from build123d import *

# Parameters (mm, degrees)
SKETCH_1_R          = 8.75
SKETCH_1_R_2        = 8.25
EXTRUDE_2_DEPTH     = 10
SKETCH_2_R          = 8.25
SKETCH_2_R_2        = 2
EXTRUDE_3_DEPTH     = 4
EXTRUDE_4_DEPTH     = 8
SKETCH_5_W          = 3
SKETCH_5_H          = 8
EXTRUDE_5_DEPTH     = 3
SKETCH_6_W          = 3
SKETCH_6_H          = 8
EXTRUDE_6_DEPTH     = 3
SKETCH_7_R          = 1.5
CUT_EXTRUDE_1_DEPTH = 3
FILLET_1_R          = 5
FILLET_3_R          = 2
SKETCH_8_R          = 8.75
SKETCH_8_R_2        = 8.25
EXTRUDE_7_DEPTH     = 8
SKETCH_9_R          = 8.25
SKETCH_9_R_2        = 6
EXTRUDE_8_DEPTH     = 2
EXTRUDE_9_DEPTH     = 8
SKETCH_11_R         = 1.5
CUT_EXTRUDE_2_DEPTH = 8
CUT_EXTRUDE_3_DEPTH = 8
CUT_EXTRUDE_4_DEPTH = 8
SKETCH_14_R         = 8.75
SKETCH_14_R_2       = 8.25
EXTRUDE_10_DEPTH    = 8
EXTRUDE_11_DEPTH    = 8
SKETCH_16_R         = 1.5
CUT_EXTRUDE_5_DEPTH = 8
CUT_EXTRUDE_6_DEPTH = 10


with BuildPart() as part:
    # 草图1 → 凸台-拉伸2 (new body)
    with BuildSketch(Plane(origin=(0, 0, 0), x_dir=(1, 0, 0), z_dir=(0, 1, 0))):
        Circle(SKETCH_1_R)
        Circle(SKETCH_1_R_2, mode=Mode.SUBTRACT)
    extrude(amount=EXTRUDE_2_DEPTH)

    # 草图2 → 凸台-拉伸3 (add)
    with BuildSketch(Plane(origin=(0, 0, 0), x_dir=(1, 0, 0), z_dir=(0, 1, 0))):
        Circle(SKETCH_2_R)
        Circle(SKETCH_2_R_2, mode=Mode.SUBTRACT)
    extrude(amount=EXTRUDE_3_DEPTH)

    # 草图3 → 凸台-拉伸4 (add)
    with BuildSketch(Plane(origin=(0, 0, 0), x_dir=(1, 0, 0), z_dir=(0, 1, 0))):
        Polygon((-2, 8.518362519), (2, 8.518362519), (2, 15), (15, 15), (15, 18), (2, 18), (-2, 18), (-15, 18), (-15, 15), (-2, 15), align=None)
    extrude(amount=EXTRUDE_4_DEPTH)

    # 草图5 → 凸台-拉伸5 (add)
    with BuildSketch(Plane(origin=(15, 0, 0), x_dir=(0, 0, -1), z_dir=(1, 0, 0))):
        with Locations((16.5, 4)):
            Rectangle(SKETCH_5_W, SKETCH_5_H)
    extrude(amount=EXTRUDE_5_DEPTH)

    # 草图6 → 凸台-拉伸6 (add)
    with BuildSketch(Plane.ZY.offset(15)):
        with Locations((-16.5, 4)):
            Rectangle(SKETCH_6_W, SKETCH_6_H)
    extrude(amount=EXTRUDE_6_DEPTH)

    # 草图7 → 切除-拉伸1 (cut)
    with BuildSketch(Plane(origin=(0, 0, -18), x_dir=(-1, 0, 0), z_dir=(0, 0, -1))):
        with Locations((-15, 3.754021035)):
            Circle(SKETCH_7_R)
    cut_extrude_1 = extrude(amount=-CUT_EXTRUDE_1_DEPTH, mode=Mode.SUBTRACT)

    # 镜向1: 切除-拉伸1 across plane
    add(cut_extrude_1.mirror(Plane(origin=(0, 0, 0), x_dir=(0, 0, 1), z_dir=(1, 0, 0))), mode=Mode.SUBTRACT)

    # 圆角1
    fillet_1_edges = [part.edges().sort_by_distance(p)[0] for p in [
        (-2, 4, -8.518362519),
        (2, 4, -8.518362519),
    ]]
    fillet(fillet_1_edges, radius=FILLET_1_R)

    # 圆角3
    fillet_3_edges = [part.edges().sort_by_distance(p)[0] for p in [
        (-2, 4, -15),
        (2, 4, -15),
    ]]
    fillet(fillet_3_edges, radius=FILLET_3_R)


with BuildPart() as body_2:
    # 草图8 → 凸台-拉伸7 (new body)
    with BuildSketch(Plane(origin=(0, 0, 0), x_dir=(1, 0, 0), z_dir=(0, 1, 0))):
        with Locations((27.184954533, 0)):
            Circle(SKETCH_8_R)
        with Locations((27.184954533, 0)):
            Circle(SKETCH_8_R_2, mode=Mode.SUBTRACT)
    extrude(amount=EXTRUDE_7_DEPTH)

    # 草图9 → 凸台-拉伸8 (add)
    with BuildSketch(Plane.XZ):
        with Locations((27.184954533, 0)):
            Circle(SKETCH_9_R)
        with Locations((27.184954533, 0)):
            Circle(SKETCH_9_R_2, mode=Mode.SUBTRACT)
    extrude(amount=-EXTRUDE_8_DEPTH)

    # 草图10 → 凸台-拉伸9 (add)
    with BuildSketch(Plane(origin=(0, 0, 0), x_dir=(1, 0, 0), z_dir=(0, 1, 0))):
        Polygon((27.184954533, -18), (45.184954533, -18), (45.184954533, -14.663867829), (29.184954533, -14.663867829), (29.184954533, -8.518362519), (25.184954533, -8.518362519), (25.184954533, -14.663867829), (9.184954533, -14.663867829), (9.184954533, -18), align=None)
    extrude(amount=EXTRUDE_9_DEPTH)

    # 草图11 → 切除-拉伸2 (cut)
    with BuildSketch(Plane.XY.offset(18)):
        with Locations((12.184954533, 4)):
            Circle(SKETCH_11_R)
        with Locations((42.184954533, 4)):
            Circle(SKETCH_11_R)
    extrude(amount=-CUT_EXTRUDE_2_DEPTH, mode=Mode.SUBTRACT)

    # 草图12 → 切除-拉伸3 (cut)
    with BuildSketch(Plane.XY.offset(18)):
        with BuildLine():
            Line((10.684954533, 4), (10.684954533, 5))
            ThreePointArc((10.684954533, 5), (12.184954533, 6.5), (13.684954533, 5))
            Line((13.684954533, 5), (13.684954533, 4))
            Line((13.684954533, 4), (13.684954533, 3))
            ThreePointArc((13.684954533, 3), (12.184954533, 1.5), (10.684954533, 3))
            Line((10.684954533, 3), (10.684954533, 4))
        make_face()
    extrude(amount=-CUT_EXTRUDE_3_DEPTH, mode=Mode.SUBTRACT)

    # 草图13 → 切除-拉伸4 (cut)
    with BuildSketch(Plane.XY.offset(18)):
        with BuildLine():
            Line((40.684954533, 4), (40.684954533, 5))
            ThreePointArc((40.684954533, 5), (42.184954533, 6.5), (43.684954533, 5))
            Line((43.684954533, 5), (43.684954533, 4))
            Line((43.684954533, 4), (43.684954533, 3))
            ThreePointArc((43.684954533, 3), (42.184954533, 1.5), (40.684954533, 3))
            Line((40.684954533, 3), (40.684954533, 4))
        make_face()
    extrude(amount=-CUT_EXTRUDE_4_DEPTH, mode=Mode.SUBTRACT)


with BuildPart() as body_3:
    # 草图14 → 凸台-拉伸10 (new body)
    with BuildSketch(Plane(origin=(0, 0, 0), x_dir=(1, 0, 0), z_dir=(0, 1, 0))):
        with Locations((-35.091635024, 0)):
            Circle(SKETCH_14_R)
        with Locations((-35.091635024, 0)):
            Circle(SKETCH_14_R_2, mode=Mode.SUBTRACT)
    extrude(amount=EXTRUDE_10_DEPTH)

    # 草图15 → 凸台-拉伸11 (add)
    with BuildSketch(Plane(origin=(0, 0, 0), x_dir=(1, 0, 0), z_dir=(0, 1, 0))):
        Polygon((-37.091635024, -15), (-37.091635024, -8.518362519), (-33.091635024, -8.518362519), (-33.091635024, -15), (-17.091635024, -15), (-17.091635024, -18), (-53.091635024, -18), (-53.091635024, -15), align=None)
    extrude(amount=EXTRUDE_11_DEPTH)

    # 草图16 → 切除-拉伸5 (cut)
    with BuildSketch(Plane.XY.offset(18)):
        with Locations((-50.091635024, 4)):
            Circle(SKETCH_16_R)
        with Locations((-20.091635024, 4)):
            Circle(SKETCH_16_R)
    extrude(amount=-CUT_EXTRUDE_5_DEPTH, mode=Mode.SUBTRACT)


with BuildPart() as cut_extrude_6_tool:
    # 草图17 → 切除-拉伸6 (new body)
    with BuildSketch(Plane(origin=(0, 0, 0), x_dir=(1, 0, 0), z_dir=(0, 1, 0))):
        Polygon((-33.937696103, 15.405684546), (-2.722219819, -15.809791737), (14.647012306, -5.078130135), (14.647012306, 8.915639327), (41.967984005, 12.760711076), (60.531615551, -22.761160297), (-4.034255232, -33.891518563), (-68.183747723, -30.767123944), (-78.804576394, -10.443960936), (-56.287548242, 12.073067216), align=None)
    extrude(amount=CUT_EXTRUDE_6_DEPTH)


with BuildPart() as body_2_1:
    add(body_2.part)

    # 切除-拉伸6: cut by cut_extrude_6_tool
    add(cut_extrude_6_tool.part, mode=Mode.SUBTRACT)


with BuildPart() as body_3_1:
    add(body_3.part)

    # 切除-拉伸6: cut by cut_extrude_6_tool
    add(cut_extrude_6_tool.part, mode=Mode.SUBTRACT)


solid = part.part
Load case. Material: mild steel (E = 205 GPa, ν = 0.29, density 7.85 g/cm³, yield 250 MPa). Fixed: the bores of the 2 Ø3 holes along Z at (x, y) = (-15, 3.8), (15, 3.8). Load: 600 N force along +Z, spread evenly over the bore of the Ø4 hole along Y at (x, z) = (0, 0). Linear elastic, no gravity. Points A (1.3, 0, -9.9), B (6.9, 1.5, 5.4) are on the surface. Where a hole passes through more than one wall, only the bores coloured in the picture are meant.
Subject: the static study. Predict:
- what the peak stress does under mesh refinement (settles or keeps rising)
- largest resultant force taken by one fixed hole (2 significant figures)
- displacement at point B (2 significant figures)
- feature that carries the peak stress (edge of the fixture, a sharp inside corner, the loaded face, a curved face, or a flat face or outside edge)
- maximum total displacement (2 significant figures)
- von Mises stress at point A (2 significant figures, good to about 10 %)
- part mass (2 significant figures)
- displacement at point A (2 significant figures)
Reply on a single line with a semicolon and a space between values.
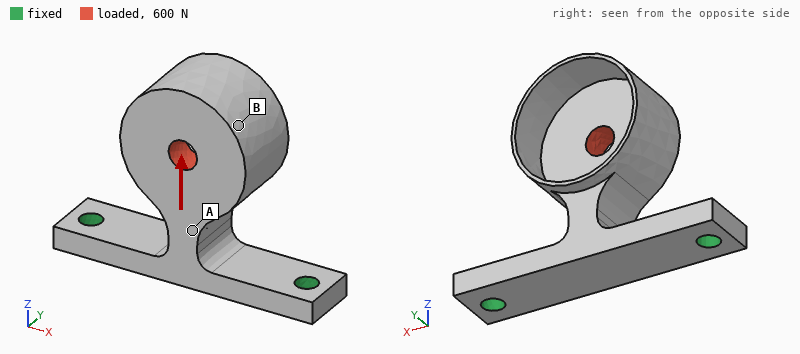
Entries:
keeps rising; 320 N; 41 µm; edge of the fixture; 47 µm; 36 MPa; 17 g; 24 µm
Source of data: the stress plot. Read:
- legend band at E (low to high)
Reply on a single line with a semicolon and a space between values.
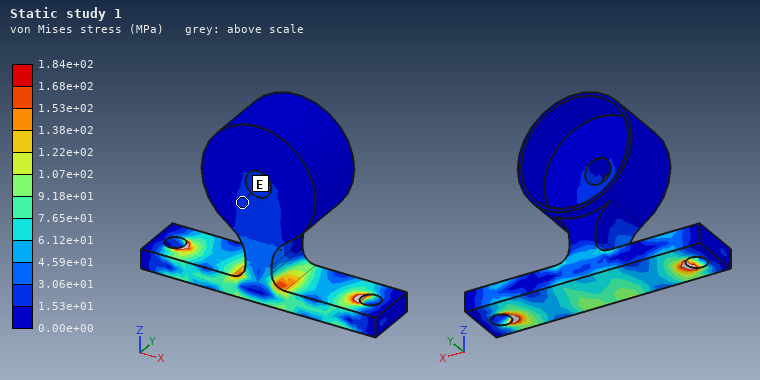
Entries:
1.53e+01 to 3.06e+01 MPa
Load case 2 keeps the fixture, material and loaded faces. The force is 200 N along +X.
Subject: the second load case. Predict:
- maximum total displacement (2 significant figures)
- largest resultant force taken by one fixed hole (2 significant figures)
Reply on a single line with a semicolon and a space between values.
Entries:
67 µm; 200 N
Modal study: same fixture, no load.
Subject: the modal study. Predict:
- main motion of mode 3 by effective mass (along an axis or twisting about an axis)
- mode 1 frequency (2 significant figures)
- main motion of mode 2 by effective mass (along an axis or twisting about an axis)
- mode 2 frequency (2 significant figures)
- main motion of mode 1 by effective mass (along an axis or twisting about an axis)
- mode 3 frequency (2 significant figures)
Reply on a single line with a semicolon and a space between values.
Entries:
along Z; 2500 Hz; along X; 3400 Hz; along Y; 8500 Hz
